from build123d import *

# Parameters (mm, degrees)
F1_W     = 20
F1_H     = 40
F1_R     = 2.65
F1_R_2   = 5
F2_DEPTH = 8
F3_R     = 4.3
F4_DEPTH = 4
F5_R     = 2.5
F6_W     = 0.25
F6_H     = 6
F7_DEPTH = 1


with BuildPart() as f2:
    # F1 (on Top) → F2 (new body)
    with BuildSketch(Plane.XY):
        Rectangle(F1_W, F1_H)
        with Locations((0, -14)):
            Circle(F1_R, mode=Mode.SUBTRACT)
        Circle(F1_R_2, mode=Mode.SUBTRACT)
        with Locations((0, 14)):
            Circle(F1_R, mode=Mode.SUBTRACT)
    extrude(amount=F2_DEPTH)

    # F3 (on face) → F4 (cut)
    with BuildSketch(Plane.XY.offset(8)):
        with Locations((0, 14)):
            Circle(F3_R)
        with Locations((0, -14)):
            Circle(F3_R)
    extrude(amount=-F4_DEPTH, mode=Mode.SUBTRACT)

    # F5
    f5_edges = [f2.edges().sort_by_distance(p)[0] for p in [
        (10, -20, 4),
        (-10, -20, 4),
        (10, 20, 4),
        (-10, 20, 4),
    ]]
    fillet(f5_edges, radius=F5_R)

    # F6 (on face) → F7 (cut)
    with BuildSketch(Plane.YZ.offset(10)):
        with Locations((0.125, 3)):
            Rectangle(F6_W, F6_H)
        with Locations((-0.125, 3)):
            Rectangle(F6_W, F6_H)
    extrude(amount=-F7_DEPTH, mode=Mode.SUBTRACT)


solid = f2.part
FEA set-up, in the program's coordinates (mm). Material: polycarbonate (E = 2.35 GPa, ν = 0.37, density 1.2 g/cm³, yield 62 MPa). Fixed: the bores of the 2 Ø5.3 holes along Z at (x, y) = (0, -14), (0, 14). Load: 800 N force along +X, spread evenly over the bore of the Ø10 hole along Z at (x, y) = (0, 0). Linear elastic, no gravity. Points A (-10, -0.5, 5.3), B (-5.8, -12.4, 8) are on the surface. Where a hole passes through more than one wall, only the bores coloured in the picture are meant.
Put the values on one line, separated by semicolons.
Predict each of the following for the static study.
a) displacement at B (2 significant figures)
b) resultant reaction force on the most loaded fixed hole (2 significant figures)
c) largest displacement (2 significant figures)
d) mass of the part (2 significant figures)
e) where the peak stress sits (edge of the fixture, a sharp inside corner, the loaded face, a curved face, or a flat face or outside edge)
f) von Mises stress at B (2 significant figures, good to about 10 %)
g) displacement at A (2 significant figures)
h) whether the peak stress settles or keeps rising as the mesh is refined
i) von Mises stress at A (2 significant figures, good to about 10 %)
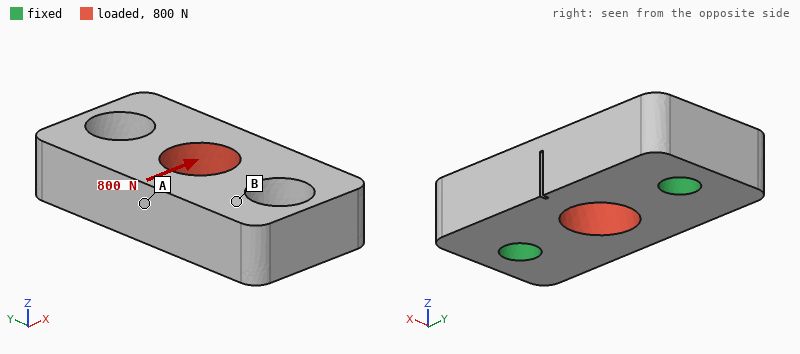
0.055 mm; 400 N; 0.12 mm; 6.1 g; edge of the fixture; 3.9 MPa; 0.10 mm; keeps rising; 9.4 MPa
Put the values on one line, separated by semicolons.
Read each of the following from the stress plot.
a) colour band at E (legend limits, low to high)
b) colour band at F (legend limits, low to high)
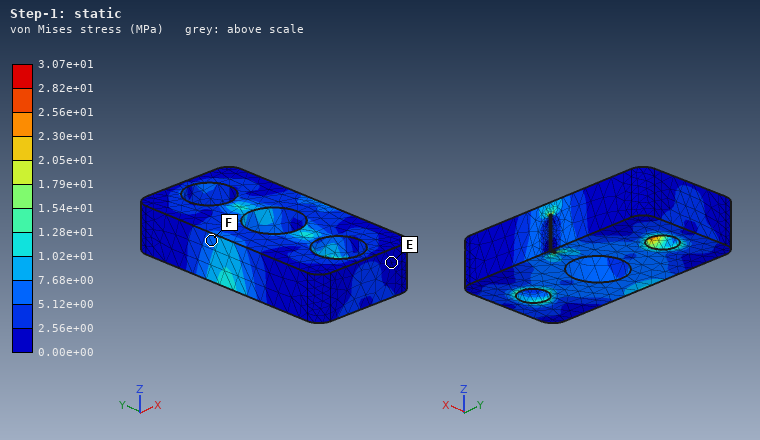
0.00e+00 to 2.56e+00 MPa; 5.12e+00 to 7.68e+00 MPa
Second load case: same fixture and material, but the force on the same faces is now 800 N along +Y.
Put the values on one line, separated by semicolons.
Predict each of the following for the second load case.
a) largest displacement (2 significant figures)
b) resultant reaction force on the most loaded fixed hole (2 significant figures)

33 µm; 400 N
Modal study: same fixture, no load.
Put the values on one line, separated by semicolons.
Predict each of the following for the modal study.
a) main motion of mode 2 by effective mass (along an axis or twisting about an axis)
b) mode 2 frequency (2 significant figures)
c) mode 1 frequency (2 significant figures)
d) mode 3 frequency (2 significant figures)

along Z; 7600 Hz; 5600 Hz; 9100 Hz
